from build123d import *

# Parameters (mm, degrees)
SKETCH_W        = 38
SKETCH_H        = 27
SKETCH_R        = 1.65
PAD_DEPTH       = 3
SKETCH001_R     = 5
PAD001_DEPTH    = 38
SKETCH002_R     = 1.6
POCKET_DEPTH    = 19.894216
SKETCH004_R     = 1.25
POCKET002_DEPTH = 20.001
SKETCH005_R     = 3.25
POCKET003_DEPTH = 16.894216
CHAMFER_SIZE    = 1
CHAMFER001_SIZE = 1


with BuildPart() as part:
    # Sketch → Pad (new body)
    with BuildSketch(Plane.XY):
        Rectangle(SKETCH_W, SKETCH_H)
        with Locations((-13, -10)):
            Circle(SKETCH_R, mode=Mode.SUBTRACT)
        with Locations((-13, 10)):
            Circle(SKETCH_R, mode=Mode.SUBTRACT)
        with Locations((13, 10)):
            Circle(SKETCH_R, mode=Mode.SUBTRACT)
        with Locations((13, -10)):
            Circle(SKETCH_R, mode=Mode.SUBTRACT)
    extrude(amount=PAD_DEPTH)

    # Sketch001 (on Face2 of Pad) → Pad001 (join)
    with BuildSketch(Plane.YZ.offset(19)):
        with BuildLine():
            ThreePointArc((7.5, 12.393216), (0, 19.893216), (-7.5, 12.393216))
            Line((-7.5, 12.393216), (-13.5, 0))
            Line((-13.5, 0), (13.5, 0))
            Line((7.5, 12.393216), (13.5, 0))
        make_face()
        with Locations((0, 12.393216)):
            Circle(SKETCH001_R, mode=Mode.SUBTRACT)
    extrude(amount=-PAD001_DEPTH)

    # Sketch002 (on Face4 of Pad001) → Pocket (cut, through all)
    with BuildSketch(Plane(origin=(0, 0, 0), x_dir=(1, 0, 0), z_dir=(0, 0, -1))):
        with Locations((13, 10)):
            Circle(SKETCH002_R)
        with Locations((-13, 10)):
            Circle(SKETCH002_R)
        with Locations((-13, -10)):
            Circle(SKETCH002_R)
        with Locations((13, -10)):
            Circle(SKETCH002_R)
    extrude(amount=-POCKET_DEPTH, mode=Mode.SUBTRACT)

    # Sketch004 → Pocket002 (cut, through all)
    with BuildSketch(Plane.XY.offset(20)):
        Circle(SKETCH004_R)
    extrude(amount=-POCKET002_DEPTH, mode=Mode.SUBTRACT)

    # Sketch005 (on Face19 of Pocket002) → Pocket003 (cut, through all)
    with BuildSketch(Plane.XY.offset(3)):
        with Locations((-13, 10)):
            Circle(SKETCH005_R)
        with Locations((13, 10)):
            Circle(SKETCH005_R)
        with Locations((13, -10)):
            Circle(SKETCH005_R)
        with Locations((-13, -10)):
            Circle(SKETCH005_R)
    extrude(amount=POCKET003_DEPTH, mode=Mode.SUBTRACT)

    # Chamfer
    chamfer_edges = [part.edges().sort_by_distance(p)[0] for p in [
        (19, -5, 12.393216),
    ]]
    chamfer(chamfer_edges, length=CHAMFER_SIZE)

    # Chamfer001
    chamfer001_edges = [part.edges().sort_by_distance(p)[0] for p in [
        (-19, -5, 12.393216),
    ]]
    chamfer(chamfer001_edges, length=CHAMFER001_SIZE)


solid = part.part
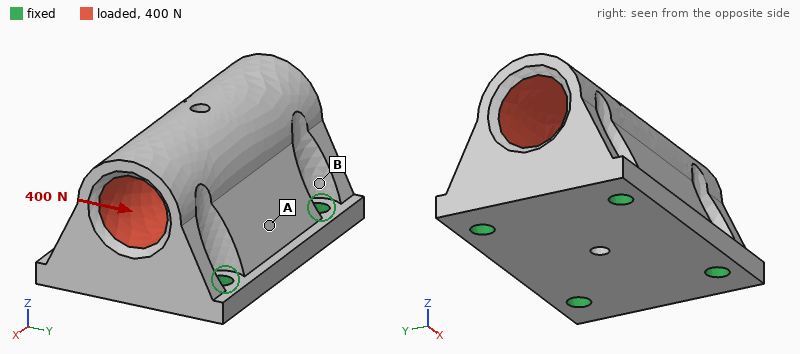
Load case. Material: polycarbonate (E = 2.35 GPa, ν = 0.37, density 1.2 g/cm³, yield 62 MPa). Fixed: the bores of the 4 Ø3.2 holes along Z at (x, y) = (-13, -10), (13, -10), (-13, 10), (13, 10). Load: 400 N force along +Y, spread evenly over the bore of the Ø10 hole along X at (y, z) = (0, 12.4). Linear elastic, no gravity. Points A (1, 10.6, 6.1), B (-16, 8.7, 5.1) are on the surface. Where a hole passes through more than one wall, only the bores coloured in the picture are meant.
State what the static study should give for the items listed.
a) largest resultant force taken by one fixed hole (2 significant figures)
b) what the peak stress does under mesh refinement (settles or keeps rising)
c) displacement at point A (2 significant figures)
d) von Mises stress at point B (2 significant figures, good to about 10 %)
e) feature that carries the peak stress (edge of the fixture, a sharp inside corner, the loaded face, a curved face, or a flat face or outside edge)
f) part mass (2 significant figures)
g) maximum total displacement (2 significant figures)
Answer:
150 N
keeps rising
33 µm
4.2 MPa
edge of the fixture
12 g
79 µm
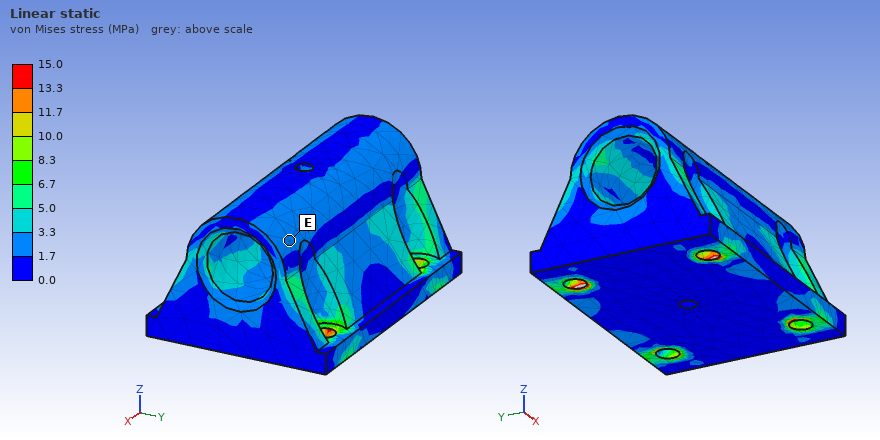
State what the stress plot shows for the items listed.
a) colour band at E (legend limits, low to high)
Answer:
1.7 to 3.3 MPa
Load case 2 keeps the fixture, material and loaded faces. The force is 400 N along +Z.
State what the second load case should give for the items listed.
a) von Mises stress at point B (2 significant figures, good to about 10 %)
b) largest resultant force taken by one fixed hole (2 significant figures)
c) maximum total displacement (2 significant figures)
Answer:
3.0 MPa
110 N
27 µm
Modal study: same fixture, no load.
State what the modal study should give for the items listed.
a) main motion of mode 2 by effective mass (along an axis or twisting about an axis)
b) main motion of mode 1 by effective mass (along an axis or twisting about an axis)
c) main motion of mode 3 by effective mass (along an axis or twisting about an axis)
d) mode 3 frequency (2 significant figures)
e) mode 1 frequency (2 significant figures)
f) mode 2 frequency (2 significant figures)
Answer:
along X
along Y
along Z
7000 Hz
5600 Hz
6400 Hz
